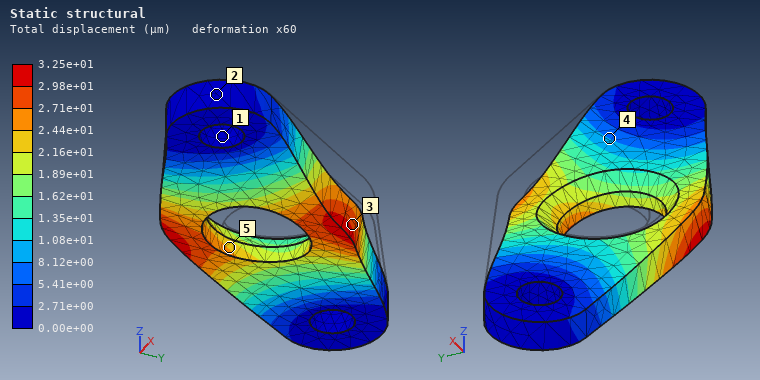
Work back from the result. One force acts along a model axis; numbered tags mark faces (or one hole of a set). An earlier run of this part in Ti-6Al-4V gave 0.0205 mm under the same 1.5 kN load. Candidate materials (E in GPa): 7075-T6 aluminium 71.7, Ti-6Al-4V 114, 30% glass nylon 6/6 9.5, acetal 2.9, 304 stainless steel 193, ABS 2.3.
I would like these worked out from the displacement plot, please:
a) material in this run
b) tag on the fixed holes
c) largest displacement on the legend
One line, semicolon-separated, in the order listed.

7075-T6 aluminium; 1; 3.25e+01 µm
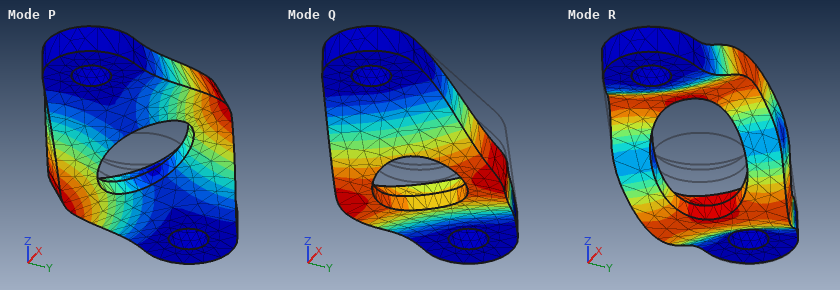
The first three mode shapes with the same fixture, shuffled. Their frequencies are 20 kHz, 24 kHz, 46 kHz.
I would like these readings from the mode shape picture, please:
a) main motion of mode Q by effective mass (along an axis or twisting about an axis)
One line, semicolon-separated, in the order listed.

along Z
